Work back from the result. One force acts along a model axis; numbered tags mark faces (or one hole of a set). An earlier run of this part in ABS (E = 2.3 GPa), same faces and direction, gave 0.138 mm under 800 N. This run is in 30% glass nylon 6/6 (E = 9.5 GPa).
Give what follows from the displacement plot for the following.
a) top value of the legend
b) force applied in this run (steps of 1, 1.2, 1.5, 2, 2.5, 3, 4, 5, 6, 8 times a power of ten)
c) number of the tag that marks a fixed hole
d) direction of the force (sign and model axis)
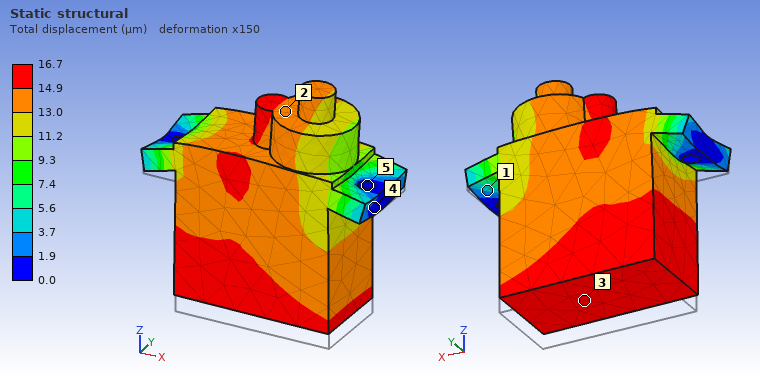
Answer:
16.7 µm
400 N
5
+Z
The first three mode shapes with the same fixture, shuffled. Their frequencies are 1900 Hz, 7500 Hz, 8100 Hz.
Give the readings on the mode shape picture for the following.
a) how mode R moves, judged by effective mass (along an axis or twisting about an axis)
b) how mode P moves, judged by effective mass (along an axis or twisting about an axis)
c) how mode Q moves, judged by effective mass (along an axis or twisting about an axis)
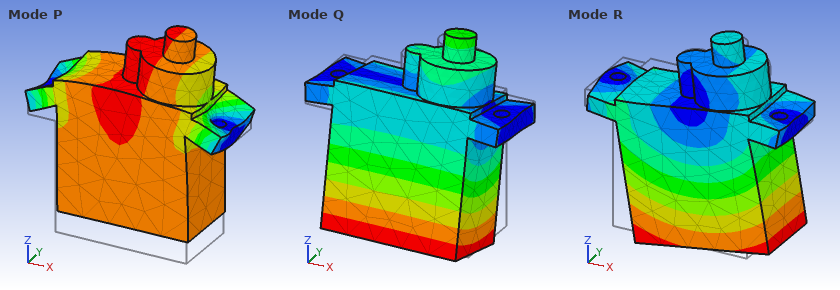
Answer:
along X
along Z
along Y
